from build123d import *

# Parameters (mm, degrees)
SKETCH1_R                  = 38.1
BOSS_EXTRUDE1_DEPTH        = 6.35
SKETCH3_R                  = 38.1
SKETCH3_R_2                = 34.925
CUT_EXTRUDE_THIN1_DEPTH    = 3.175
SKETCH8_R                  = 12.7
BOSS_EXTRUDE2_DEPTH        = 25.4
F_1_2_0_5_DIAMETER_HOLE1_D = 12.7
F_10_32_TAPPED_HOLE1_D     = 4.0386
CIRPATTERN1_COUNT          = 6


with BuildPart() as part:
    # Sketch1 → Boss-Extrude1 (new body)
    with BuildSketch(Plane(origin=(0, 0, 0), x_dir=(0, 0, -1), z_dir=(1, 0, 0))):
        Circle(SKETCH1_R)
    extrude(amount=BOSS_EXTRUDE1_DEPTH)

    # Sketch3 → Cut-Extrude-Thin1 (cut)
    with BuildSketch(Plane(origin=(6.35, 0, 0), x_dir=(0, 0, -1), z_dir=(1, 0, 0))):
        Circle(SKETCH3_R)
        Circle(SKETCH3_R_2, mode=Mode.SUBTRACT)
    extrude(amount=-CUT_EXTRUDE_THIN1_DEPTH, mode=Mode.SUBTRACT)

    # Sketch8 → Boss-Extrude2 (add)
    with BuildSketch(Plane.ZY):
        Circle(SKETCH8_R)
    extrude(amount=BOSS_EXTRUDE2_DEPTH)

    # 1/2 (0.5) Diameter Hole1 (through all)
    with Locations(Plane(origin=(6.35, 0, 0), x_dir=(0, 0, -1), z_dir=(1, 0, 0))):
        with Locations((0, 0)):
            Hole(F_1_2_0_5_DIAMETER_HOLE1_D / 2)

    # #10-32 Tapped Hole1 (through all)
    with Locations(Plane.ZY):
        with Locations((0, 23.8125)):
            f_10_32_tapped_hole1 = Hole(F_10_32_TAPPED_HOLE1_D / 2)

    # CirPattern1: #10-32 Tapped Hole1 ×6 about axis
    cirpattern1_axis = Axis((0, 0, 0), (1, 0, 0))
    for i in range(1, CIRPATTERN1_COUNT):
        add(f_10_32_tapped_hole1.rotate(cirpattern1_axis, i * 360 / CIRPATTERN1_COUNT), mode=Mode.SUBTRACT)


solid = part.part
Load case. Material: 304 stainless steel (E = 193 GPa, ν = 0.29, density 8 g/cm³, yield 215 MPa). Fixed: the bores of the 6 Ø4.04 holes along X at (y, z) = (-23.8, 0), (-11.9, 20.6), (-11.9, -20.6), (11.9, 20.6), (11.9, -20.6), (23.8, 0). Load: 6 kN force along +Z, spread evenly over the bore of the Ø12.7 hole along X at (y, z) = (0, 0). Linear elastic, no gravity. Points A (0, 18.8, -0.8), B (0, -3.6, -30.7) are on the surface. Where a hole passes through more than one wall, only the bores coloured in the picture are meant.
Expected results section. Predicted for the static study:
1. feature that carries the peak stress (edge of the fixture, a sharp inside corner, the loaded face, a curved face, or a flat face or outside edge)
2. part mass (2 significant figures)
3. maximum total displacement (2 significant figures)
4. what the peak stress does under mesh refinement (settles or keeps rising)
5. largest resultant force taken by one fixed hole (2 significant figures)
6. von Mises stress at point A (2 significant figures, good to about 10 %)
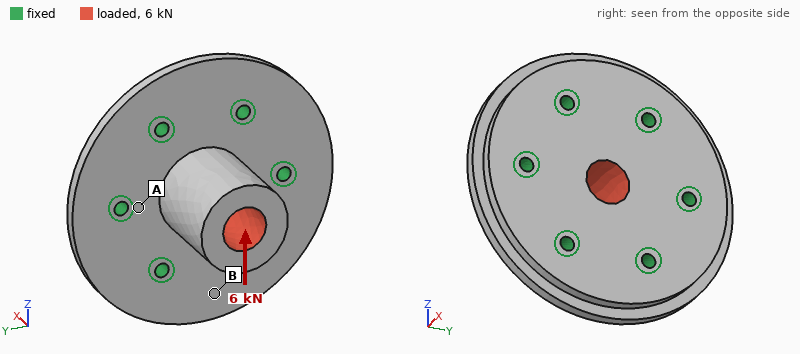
edge of the fixture
280 g
19 µm
keeps rising
1.7 kN
22 MPa
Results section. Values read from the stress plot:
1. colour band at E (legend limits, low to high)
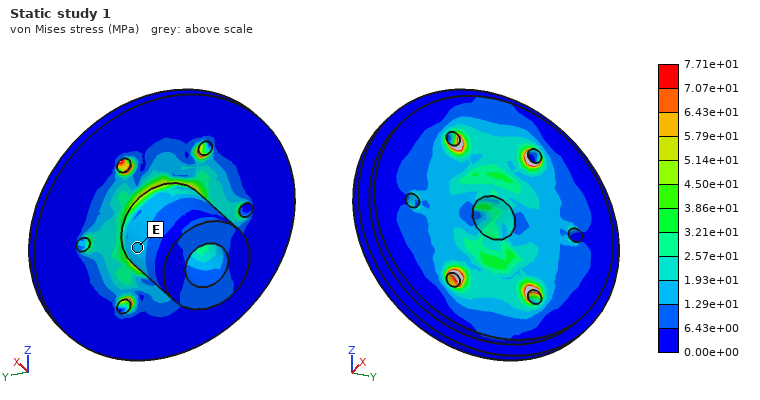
1.29e+01 to 1.93e+01 MPa
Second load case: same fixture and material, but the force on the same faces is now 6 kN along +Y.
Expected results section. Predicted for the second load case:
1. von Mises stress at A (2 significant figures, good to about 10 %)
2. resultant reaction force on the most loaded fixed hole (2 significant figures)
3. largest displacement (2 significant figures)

14 MPa
2.0 kN
19 µm
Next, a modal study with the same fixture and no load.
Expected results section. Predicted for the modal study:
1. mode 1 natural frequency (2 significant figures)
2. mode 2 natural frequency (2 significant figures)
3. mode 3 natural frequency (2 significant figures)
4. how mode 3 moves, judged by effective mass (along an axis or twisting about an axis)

11 kHz
11 kHz
15 kHz
along X
